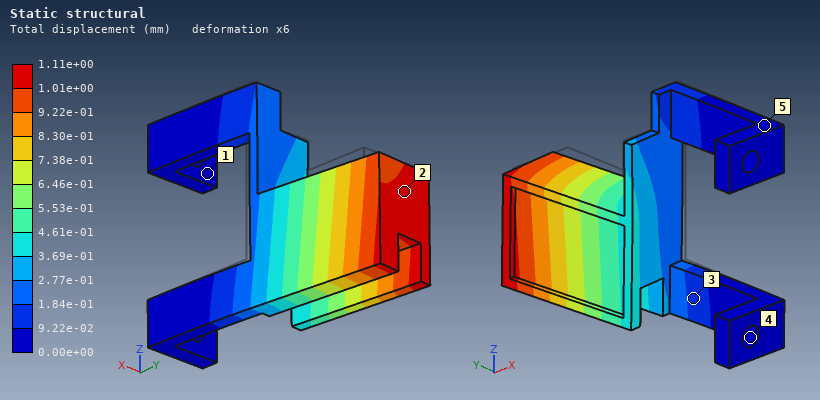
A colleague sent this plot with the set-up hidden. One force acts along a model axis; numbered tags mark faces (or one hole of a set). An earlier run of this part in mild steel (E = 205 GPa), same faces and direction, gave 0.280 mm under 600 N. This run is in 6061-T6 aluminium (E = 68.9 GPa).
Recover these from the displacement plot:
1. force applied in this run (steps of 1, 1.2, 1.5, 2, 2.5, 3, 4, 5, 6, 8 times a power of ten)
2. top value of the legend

800 N
1.11e+00 mm
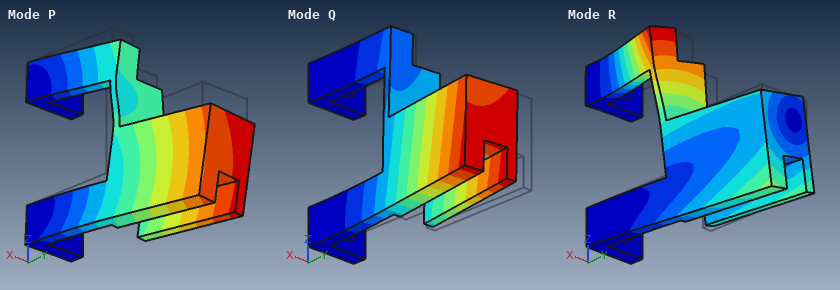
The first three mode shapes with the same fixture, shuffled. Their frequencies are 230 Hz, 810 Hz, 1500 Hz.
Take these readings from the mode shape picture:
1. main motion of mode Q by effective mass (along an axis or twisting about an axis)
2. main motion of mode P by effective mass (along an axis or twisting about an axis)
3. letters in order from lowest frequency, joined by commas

along X
along Z
Q, P, R
